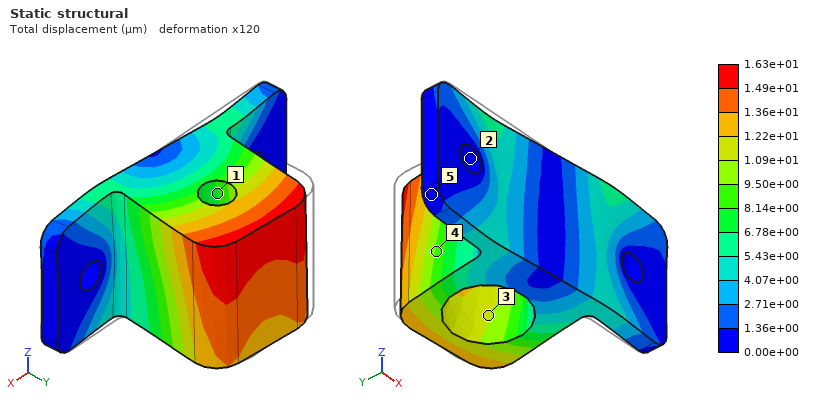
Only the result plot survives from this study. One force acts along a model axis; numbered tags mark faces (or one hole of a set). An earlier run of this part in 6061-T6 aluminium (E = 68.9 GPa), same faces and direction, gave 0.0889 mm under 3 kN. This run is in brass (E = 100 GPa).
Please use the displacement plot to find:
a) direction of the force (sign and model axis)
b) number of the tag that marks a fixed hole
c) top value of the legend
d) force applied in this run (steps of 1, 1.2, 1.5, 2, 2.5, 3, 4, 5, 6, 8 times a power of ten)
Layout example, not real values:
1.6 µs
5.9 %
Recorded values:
+X
2
1.63e+01 µm
800 N
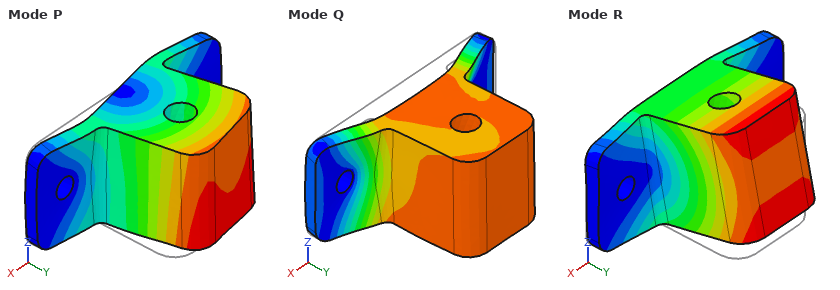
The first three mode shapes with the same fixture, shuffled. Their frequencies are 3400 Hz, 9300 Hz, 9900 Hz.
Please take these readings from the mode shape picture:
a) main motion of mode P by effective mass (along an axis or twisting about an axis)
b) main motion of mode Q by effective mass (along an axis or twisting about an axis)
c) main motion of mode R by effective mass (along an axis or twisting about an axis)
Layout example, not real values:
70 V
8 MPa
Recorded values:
along X
along Y
along Z
